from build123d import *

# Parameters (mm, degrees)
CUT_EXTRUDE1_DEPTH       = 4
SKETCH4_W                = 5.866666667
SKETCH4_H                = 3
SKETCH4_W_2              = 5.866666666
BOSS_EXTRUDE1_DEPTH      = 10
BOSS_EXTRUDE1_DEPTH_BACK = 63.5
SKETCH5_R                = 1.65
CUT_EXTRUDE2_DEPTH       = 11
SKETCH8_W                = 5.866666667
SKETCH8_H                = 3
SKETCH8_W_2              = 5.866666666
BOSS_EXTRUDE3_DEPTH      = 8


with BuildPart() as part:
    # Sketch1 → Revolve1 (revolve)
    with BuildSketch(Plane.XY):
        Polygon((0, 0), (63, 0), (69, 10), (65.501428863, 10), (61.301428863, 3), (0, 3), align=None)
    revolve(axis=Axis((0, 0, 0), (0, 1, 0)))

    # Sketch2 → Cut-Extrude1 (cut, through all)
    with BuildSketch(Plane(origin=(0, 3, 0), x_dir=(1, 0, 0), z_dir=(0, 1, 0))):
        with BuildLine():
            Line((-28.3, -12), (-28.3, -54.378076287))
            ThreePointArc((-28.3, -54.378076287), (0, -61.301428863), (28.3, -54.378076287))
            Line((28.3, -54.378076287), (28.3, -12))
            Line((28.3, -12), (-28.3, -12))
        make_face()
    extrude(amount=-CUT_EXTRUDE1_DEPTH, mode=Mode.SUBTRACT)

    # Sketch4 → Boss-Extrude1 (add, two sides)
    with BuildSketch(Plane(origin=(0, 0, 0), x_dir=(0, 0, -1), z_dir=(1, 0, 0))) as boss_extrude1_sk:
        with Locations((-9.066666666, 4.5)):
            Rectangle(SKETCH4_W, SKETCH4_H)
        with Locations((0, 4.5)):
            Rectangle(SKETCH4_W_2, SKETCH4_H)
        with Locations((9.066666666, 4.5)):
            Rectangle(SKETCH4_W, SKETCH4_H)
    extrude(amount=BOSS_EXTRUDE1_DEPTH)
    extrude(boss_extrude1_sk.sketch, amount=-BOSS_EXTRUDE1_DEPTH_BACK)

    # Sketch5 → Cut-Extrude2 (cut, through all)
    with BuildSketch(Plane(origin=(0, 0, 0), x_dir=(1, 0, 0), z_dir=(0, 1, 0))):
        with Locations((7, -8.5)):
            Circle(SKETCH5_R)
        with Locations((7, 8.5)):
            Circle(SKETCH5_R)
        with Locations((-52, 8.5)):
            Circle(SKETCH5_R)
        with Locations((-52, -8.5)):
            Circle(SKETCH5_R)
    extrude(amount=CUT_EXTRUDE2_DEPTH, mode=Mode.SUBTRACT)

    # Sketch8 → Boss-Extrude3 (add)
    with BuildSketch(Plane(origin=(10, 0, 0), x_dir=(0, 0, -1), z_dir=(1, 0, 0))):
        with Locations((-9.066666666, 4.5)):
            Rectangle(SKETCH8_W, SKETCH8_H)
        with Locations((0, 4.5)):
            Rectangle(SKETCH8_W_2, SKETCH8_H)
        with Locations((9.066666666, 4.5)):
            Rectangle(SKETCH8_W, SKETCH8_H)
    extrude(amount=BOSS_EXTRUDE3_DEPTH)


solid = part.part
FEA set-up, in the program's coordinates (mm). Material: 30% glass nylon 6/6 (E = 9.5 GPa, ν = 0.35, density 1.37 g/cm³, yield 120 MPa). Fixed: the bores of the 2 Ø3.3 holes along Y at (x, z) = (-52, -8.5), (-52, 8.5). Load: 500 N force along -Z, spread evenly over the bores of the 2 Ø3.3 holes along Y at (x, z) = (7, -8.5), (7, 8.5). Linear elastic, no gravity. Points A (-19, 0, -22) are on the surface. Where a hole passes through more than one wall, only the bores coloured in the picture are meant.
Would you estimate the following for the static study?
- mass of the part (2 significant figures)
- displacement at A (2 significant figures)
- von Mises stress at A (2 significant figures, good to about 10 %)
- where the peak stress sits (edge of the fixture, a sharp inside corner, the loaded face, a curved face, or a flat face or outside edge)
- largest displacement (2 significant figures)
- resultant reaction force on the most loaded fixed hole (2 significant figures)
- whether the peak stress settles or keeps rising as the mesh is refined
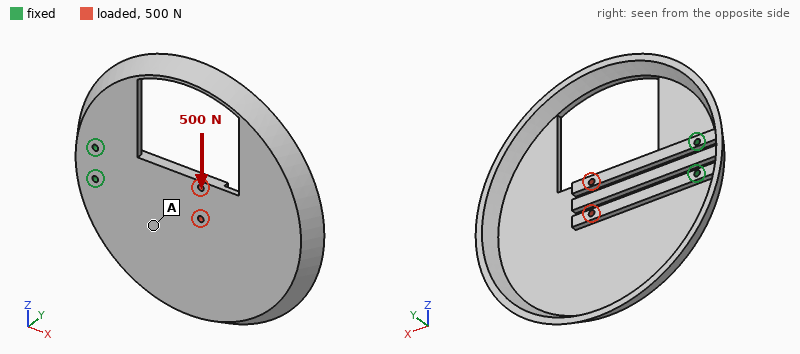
61 g
0.20 mm
4.6 MPa
edge of the fixture
0.74 mm
1.5 kN
keeps rising
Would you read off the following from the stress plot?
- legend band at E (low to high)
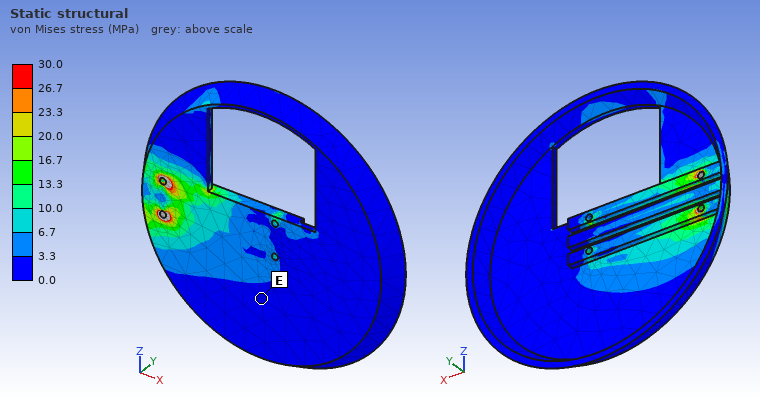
0.0 to 3.3 MPa
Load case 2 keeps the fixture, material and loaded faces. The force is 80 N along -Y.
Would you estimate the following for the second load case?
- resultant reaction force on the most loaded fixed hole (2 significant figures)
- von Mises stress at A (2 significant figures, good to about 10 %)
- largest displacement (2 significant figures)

84 N
5.3 MPa
2.3 mm
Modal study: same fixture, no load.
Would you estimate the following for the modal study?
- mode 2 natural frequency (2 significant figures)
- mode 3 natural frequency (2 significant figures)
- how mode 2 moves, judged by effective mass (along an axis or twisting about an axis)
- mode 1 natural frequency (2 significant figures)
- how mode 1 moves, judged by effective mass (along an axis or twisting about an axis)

300 Hz
630 Hz
twisting about X
150 Hz
along Y
